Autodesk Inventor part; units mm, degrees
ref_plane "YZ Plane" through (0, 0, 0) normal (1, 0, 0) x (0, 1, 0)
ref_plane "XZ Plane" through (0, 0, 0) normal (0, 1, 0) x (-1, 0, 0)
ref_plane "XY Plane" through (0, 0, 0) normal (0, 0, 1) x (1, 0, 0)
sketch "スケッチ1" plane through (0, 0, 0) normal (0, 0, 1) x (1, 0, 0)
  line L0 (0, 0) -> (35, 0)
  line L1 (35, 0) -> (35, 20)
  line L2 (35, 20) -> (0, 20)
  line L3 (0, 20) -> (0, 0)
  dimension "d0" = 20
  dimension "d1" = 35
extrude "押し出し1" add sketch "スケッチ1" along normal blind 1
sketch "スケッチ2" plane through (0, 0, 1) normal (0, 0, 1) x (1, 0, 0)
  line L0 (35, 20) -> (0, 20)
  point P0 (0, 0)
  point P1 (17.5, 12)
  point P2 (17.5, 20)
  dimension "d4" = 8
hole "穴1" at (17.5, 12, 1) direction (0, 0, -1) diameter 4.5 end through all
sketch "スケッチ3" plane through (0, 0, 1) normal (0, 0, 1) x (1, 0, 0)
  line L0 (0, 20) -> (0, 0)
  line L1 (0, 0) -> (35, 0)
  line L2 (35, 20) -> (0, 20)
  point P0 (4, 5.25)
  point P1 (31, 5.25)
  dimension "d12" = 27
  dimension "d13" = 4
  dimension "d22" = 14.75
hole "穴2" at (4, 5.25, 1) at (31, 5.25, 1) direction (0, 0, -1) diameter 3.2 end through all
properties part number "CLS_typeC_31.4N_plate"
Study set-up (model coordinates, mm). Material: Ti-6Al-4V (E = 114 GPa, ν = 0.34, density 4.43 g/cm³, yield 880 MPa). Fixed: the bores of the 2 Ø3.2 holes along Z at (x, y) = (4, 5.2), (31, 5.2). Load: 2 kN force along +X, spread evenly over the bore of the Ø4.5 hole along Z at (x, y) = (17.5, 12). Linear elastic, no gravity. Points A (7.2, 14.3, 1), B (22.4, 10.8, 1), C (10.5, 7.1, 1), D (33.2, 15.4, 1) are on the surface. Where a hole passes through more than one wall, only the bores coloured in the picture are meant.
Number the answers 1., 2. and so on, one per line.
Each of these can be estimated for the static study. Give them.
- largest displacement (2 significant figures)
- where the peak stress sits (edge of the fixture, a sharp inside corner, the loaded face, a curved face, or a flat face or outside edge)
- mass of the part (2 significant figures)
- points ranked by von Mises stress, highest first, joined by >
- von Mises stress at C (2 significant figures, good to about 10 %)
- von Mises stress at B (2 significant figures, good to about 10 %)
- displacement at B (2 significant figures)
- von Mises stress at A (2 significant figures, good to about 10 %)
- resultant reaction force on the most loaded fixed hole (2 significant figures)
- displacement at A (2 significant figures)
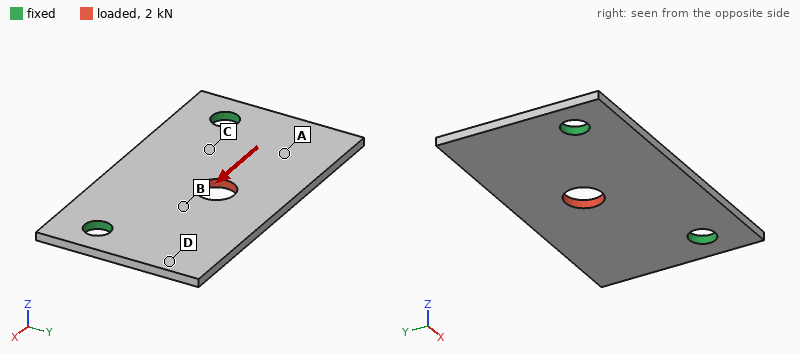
1. 21 µm
2. edge of the fixture
3. 3.0 g
4. B > C > A > D
5. 110 MPa
6. 140 MPa
7. 13 µm
8. 42 MPa
9. 1.1 kN
10. 13 µm
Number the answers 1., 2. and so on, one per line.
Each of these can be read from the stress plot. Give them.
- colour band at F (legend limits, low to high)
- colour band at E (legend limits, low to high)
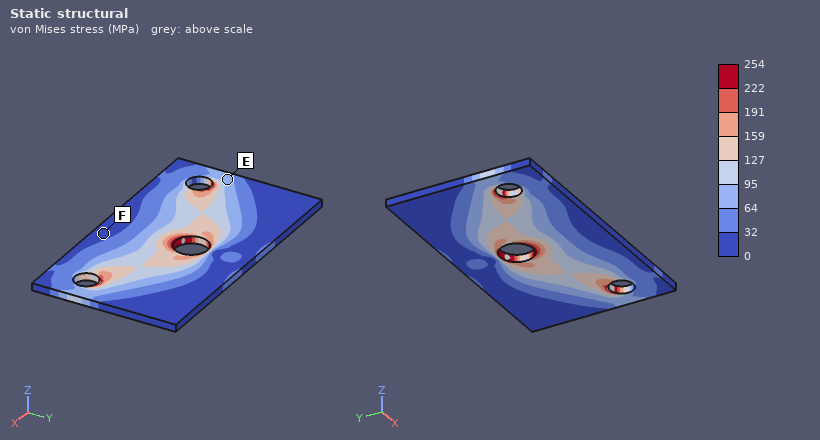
1. 0 to 32 MPa
2. 64 to 95 MPa
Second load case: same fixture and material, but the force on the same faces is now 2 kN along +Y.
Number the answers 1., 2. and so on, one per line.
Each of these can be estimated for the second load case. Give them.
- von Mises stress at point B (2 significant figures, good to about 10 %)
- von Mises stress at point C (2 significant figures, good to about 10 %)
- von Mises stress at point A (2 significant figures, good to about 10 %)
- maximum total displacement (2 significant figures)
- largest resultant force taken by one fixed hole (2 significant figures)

1. 120 MPa
2. 120 MPa
3. 73 MPa
4. 28 µm
5. 1.1 kN
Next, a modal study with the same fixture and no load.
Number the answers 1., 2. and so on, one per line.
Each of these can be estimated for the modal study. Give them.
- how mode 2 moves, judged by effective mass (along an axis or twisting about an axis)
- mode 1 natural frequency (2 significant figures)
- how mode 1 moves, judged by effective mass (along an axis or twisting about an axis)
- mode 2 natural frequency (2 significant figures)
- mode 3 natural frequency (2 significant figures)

1. twisting about Y
2. 3400 Hz
3. along Z
4. 5800 Hz
5. 7700 Hz
